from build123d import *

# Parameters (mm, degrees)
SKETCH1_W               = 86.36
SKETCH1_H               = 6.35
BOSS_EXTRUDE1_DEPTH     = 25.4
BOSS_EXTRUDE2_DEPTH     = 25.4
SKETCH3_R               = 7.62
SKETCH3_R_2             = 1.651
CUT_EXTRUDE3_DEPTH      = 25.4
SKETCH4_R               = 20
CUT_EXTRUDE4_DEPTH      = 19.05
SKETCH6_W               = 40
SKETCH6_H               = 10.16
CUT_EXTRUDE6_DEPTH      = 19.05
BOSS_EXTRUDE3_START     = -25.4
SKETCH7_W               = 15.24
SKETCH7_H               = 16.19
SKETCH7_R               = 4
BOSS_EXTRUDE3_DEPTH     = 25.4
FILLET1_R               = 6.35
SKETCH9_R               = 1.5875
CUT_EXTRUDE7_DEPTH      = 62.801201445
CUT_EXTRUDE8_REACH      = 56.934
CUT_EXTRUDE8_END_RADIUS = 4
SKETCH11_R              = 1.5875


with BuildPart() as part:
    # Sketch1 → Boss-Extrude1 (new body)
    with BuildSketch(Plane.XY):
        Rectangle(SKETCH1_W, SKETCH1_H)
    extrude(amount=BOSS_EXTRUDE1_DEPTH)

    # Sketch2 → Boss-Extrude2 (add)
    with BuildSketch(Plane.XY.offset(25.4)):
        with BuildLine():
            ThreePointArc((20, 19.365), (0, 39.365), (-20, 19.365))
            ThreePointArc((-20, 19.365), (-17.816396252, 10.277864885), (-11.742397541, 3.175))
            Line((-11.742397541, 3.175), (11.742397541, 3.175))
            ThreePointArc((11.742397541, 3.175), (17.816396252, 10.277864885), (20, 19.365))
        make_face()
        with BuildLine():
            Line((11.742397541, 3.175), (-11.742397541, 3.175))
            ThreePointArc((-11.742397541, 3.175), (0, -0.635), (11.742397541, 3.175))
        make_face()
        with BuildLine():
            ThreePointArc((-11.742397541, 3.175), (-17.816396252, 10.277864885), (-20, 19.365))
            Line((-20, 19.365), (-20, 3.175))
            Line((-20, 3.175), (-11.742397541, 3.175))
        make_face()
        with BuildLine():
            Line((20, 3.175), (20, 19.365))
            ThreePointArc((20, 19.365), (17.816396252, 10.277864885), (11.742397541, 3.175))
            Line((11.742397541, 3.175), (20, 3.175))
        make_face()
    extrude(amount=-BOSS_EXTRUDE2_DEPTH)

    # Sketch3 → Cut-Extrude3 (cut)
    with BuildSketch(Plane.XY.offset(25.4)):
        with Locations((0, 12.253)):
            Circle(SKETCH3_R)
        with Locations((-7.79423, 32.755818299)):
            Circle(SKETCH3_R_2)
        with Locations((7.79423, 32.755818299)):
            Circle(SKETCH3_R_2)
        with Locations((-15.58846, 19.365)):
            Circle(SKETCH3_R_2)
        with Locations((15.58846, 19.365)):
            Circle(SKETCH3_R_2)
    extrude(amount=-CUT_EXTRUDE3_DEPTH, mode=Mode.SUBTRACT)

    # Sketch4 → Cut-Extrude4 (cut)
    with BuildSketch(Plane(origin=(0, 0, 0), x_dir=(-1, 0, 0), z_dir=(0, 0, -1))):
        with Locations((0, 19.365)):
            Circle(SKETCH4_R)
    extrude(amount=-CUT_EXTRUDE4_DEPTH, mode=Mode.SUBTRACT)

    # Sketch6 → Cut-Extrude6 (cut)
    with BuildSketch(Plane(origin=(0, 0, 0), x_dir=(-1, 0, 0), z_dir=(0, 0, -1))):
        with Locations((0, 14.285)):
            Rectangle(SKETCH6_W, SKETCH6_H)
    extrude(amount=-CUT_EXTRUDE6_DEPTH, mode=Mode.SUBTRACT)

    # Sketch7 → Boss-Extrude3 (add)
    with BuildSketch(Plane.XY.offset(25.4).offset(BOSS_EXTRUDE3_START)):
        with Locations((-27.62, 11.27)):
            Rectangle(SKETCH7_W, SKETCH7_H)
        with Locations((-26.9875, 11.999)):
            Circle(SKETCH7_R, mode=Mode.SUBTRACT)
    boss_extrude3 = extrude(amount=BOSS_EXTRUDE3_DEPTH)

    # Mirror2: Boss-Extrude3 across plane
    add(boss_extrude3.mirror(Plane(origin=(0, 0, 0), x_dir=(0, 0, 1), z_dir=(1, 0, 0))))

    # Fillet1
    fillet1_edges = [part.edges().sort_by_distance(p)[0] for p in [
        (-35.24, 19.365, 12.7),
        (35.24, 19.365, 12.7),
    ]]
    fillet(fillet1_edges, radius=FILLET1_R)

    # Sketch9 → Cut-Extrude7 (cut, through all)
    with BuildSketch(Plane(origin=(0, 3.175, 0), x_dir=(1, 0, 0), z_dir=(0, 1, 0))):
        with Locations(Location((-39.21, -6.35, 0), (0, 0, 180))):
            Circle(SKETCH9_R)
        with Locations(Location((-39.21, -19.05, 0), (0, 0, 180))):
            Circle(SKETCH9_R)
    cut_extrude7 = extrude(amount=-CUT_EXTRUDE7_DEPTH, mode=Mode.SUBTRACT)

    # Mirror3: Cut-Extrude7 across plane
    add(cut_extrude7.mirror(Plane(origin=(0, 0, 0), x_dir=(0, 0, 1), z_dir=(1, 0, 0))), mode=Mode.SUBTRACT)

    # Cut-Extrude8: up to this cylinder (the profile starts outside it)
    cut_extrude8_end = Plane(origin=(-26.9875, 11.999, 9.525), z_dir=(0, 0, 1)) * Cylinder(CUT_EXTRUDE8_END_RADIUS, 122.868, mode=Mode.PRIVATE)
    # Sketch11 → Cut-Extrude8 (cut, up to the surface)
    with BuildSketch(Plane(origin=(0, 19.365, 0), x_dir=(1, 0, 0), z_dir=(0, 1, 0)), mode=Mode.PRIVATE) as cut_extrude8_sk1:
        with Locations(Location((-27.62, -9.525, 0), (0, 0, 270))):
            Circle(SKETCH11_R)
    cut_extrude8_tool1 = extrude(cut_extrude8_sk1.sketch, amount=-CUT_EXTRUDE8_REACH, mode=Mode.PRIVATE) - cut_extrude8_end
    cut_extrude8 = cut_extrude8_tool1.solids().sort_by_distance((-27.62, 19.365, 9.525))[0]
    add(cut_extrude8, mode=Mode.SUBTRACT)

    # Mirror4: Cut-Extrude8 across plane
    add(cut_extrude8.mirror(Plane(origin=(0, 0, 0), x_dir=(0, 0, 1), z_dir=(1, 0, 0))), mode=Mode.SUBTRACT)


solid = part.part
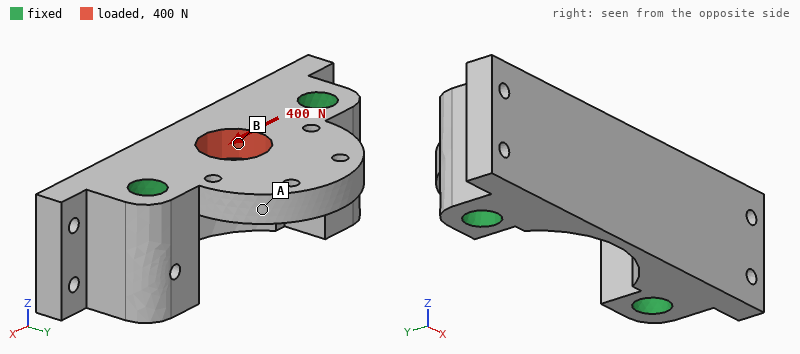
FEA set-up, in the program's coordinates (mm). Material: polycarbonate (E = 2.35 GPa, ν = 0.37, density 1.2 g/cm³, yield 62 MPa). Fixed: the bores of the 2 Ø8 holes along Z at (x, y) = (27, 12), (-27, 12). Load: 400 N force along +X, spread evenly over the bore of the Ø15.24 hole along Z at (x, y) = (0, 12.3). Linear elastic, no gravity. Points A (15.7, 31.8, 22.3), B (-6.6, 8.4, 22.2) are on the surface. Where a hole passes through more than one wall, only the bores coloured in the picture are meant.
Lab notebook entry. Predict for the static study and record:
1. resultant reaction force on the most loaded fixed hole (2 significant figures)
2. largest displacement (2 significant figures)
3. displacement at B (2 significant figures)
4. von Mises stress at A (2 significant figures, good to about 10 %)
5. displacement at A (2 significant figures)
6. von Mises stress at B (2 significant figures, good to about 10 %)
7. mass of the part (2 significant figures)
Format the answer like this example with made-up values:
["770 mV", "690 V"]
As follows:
["200 N", "20 µm", "11 µm", "0.35 MPa", "14 µm", "1.8 MPa", "36 g"]
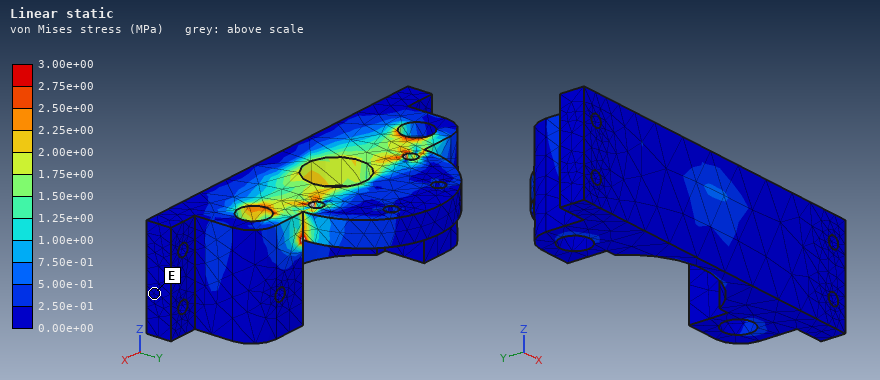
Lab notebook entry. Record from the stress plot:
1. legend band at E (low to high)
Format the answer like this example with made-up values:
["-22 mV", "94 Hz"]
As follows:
["0.00e+00 to 2.50e-01 MPa"]
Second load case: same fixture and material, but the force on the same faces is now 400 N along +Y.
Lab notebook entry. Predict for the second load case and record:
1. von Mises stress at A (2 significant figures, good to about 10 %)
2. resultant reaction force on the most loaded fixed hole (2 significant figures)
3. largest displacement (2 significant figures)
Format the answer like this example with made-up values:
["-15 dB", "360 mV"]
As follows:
["0.97 MPa", "200 N", "44 µm"]
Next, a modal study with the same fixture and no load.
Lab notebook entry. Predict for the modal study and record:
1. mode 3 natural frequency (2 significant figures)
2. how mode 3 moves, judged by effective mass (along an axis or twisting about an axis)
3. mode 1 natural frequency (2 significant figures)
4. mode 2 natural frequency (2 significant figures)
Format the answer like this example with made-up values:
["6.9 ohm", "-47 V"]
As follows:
["6200 Hz", "along Y", "1800 Hz", "4900 Hz"]
